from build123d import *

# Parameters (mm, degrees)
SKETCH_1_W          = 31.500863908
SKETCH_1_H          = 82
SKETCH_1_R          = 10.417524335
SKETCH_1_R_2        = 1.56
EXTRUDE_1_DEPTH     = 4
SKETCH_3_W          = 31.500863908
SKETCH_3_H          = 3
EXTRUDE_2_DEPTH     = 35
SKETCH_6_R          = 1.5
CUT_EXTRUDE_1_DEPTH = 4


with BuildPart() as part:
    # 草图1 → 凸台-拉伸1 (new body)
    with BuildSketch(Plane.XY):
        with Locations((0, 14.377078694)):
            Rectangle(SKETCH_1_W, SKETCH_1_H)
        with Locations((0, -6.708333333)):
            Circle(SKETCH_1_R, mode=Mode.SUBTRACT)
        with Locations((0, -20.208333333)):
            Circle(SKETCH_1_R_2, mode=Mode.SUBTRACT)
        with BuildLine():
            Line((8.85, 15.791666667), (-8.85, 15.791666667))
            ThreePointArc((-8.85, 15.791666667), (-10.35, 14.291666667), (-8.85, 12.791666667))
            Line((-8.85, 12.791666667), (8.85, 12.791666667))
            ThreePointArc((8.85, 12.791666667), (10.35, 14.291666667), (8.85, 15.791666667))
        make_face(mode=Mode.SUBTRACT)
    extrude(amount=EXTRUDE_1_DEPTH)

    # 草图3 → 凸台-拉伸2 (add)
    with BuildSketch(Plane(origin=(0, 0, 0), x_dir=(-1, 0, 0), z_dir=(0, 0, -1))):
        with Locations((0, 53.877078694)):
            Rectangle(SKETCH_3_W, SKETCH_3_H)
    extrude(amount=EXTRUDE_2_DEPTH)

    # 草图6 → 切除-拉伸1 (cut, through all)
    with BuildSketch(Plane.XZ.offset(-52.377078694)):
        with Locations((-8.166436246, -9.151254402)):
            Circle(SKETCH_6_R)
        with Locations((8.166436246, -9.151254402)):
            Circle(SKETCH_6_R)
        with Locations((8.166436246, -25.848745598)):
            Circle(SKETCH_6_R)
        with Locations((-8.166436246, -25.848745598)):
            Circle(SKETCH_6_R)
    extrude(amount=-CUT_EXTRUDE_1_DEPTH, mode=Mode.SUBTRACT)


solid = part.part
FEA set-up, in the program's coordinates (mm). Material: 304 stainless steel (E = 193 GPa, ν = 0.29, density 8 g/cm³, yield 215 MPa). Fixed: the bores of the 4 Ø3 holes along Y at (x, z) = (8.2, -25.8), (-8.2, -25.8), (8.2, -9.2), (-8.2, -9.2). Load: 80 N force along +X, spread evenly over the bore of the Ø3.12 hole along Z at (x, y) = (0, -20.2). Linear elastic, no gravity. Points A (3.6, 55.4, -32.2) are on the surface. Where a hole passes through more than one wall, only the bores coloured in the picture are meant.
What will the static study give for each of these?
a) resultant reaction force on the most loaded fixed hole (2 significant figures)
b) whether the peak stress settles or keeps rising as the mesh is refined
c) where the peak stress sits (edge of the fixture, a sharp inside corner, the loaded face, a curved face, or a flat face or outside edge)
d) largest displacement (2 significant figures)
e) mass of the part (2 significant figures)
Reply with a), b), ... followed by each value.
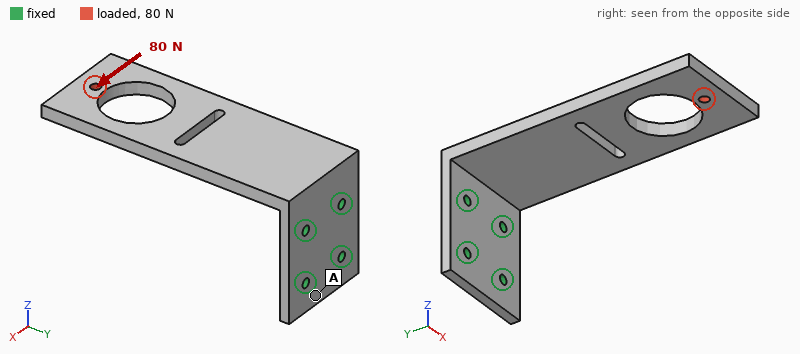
a) 320 N
b) keeps rising
c) edge of the fixture
d) 79 µm
e) 95 g
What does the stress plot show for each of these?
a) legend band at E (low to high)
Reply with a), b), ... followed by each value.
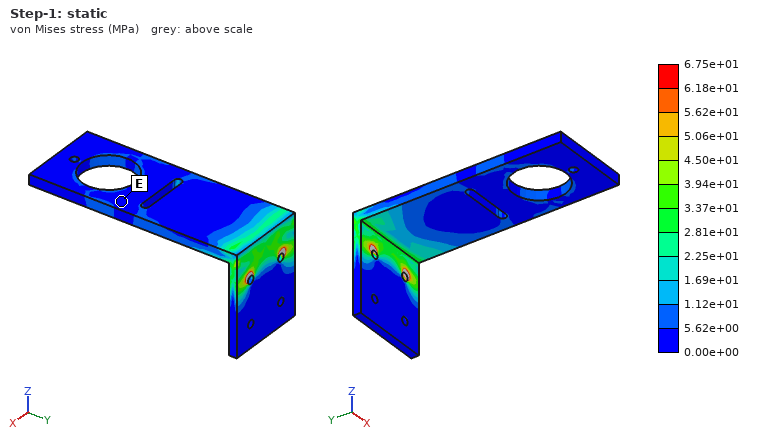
a) 0.00e+00 to 5.62e+00 MPa
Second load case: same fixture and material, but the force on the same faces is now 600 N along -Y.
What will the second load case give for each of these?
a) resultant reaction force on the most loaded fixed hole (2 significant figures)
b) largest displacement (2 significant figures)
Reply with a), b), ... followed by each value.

a) 350 N
b) 0.22 mm
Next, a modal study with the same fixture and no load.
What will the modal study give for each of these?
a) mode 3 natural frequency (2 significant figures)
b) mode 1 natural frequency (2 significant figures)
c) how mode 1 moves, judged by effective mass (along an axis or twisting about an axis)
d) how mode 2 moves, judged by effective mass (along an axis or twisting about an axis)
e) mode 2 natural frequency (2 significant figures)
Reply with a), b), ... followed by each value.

a) 1900 Hz
b) 380 Hz
c) along Z
d) along X
e) 1100 Hz
